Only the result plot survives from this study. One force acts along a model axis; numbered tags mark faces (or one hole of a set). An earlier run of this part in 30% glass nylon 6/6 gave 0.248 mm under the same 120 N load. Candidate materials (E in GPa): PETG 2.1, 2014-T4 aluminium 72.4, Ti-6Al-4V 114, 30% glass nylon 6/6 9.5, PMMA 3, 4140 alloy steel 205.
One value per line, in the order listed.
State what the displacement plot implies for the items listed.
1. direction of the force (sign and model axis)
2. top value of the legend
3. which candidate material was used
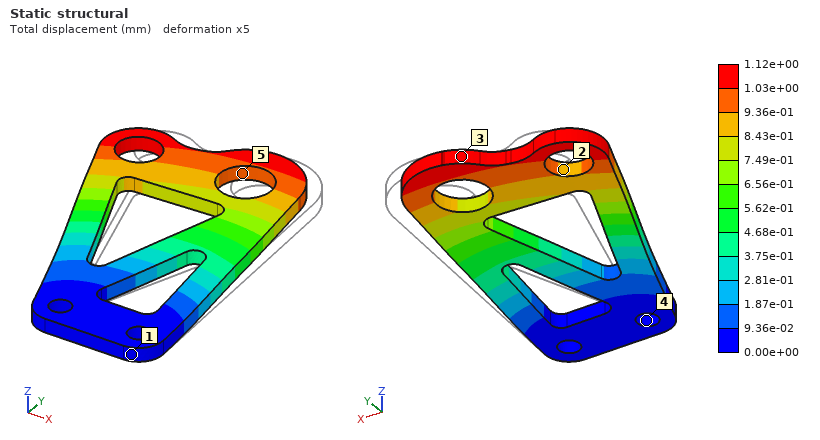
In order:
-X
1.12e+00 mm
PETG
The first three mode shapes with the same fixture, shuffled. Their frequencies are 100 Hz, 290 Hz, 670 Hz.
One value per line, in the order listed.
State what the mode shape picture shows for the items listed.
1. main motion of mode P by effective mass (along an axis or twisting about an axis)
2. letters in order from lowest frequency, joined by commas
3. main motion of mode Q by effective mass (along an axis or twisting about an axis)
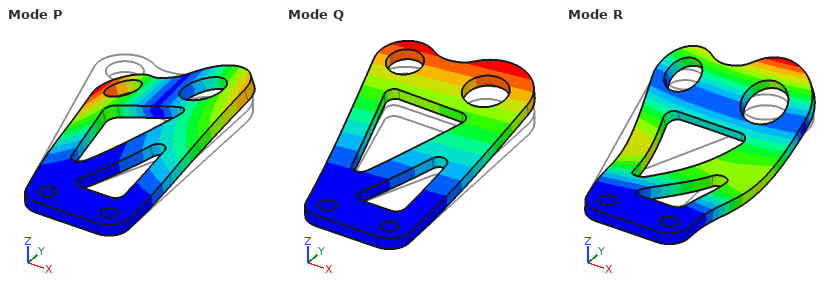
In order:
twisting about Y
Q, P, R
along Z
